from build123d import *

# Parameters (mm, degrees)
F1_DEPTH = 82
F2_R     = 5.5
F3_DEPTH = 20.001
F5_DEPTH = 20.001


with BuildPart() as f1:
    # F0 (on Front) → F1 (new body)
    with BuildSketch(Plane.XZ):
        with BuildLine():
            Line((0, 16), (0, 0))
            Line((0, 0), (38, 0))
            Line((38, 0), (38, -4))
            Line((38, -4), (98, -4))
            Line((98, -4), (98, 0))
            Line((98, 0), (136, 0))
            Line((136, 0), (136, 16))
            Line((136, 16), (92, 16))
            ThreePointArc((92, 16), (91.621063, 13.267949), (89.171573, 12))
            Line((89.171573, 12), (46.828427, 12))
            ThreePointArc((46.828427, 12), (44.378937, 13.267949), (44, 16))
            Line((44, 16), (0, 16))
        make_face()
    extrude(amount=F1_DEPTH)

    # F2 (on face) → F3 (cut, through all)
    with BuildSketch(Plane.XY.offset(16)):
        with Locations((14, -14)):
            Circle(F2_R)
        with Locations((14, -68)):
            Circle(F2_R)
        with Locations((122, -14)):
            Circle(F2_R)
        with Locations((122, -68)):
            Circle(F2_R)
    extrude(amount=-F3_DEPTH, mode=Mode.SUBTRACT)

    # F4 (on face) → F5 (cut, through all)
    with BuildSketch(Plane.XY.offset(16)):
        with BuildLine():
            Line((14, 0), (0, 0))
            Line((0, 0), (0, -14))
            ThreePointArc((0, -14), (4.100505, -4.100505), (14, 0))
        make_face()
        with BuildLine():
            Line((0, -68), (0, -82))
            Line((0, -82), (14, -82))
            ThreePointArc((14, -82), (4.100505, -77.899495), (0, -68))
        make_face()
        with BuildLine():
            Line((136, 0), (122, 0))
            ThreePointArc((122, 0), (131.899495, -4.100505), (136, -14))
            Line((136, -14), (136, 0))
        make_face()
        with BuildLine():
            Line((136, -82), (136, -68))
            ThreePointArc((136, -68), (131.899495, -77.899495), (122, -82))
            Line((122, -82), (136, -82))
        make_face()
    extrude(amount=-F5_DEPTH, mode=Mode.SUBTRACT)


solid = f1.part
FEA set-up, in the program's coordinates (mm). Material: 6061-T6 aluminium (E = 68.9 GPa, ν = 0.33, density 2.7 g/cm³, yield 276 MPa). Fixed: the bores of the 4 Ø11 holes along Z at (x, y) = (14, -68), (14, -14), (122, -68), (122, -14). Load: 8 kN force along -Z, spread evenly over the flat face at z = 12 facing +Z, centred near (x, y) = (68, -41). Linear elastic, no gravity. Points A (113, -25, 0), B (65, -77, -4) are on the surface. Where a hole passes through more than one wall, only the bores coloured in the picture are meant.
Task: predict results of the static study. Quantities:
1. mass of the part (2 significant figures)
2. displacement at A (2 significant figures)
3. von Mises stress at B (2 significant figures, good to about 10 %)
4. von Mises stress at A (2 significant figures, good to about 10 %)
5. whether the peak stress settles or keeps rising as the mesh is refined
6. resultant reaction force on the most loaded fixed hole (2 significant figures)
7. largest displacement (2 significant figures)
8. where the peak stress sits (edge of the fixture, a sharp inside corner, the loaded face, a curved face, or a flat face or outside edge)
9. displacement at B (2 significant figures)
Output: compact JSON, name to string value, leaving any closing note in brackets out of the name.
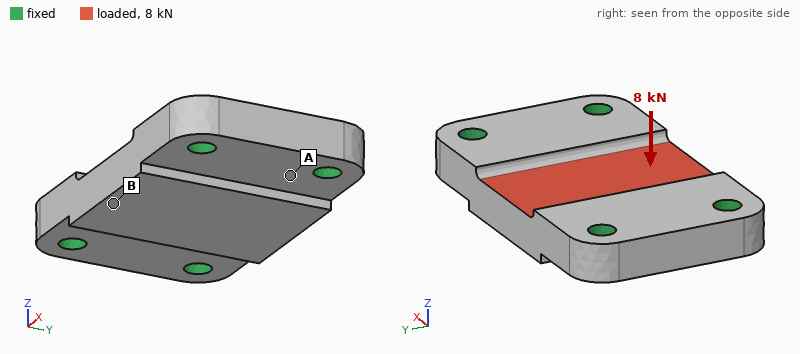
{"mass of the part": "470 g", "displacement at A": "4.6 µm", "von Mises stress at B": "22 MPa", "von Mises stress at A": "9.6 MPa", "whether the peak stress settles or keeps rising as the mesh is refined": "keeps rising", "resultant reaction force on the most loaded fixed hole": "2.6 kN", "largest displacement": "28 µm", "where the peak stress sits": "edge of the fixture", "displacement at B": "26 µm"}
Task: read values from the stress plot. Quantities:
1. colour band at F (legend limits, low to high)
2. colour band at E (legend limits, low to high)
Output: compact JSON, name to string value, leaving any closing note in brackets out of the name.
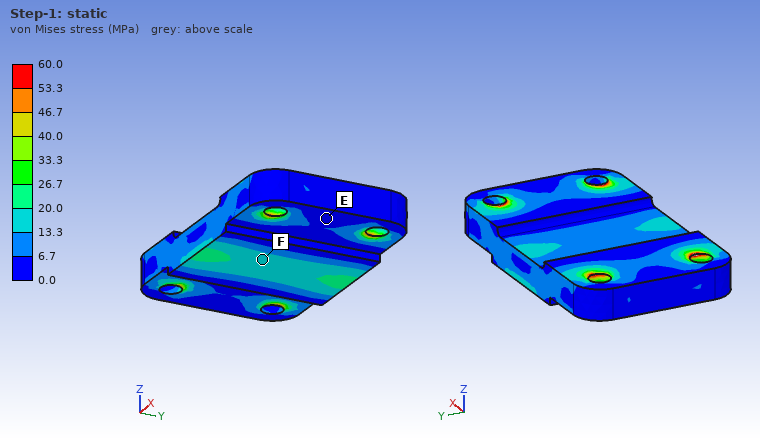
{"colour band at F": "13.3 to 20.0 MPa", "colour band at E": "0.0 to 6.7 MPa"}
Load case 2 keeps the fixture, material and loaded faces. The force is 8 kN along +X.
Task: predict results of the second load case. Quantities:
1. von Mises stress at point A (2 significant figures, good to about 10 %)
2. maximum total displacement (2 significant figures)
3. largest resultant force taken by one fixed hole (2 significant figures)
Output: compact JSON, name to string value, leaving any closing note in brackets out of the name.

{"von Mises stress at point A": "4.1 MPa", "maximum total displacement": "3.6 µm", "largest resultant force taken by one fixed hole": "2.0 kN"}
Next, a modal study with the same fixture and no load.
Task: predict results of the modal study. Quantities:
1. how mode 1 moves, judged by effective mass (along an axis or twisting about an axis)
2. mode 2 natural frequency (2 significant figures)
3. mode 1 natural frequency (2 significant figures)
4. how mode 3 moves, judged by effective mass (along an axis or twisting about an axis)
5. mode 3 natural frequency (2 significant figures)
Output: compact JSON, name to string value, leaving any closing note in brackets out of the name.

{"how mode 1 moves, judged by effective mass": "along Z", "mode 2 natural frequency": "8400 Hz", "mode 1 natural frequency": "6500 Hz", "how mode 3 moves, judged by effective mass": "along Y", "mode 3 natural frequency": "12 kHz"}
